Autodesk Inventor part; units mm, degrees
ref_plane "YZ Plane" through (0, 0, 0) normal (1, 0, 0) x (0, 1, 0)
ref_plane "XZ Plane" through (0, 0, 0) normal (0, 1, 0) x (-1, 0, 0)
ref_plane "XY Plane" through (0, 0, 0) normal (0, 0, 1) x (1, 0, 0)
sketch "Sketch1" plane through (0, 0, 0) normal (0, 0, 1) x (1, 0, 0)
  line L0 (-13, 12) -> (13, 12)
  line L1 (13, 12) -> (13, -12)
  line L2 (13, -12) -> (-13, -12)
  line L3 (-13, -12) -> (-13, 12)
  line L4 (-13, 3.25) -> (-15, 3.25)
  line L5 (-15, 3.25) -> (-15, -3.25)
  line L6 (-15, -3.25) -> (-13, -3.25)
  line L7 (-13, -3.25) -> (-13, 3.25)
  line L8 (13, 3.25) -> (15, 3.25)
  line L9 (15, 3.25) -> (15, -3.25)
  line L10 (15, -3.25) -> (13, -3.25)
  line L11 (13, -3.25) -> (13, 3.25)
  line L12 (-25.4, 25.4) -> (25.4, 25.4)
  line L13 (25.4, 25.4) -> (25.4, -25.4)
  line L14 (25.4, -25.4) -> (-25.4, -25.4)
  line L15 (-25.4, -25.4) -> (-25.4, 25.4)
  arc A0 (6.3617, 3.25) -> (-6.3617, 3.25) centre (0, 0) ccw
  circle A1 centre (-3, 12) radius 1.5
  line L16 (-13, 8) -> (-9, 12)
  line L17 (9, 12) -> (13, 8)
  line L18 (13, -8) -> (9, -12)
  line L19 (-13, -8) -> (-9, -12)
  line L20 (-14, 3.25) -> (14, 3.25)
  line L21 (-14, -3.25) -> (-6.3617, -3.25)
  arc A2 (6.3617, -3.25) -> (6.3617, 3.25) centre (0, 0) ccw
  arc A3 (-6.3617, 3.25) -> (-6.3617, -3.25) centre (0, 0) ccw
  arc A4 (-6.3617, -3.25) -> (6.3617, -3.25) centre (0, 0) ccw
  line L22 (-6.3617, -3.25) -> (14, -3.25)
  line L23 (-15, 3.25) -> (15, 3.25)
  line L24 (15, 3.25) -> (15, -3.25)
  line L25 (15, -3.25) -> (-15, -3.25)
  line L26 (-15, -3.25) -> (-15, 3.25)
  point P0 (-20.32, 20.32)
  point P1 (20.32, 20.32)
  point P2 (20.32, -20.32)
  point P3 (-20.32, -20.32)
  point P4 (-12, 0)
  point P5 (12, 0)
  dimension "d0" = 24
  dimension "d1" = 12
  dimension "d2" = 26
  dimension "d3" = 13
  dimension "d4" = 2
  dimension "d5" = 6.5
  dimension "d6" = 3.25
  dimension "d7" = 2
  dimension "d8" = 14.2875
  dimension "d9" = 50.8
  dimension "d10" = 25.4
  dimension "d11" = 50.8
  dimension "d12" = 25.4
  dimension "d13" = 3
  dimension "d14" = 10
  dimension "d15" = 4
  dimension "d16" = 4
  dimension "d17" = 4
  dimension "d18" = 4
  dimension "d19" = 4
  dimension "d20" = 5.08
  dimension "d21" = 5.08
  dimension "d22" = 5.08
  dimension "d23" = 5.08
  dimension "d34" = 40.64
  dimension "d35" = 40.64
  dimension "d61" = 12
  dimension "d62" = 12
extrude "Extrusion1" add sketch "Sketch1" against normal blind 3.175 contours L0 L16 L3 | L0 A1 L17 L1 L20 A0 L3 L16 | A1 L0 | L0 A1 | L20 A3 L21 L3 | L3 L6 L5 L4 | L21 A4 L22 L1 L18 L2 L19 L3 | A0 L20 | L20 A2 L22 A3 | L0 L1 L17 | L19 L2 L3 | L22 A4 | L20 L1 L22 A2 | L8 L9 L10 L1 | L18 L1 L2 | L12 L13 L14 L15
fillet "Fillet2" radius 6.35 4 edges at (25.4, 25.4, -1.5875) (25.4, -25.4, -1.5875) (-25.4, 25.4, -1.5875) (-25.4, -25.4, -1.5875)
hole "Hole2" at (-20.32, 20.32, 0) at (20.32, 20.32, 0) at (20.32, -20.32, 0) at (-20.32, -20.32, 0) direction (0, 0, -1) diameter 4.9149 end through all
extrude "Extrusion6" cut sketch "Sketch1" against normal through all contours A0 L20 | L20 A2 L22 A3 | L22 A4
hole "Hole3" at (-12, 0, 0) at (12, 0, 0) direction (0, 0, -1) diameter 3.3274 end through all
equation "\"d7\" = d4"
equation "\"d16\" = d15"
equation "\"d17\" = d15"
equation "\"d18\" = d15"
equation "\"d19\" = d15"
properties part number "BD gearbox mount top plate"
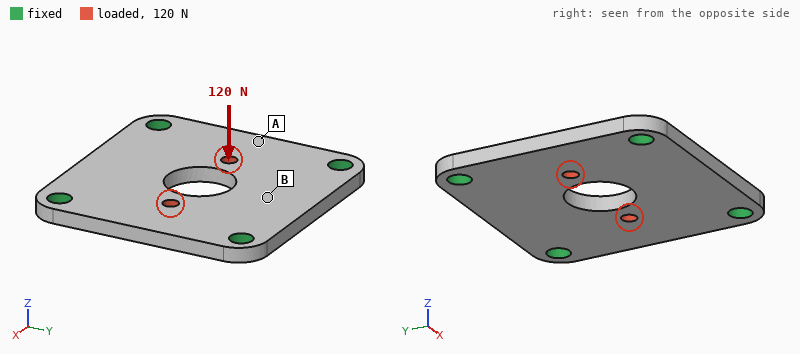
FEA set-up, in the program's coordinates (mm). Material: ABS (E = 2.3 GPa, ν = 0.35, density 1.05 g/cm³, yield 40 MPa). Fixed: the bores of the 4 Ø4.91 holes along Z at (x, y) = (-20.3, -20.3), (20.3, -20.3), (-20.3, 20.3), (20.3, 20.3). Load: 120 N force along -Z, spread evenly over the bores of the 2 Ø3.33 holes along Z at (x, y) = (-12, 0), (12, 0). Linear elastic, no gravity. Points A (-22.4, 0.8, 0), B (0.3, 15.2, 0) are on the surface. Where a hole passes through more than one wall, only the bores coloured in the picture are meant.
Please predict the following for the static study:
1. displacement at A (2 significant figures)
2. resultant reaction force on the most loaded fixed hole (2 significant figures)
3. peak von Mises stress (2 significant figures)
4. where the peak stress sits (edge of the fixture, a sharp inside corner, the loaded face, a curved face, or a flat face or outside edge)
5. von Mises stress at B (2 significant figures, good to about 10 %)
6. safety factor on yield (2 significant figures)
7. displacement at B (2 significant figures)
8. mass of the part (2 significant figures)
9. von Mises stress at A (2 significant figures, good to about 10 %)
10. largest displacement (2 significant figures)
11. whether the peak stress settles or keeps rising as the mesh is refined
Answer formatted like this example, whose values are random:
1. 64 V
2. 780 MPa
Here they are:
1. 0.12 mm
2. 30 N
3. 30 MPa
4. the loaded face
5. 2.9 MPa
6. 1.3
7. 0.13 mm
8. 7.6 g
9. 5.8 MPa
10. 0.33 mm
11. settles
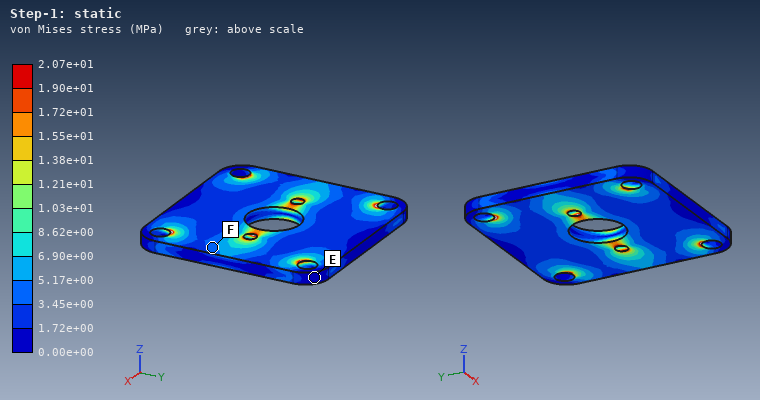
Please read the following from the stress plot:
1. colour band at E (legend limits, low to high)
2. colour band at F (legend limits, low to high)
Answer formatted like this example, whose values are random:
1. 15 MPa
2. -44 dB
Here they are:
1. 0.00e+00 to 1.72e+00 MPa
2. 3.45e+00 to 5.17e+00 MPa
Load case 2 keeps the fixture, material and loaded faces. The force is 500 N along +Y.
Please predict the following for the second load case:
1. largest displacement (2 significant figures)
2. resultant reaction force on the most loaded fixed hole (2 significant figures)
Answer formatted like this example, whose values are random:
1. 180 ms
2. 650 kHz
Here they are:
1. 39 µm
2. 130 N
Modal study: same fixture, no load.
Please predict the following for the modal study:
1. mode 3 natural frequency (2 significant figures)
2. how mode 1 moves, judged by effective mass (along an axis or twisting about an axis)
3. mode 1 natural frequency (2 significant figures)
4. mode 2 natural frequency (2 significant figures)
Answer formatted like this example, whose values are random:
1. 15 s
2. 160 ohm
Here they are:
1. 3500 Hz
2. along Z
3. 2300 Hz
4. 3400 Hz
